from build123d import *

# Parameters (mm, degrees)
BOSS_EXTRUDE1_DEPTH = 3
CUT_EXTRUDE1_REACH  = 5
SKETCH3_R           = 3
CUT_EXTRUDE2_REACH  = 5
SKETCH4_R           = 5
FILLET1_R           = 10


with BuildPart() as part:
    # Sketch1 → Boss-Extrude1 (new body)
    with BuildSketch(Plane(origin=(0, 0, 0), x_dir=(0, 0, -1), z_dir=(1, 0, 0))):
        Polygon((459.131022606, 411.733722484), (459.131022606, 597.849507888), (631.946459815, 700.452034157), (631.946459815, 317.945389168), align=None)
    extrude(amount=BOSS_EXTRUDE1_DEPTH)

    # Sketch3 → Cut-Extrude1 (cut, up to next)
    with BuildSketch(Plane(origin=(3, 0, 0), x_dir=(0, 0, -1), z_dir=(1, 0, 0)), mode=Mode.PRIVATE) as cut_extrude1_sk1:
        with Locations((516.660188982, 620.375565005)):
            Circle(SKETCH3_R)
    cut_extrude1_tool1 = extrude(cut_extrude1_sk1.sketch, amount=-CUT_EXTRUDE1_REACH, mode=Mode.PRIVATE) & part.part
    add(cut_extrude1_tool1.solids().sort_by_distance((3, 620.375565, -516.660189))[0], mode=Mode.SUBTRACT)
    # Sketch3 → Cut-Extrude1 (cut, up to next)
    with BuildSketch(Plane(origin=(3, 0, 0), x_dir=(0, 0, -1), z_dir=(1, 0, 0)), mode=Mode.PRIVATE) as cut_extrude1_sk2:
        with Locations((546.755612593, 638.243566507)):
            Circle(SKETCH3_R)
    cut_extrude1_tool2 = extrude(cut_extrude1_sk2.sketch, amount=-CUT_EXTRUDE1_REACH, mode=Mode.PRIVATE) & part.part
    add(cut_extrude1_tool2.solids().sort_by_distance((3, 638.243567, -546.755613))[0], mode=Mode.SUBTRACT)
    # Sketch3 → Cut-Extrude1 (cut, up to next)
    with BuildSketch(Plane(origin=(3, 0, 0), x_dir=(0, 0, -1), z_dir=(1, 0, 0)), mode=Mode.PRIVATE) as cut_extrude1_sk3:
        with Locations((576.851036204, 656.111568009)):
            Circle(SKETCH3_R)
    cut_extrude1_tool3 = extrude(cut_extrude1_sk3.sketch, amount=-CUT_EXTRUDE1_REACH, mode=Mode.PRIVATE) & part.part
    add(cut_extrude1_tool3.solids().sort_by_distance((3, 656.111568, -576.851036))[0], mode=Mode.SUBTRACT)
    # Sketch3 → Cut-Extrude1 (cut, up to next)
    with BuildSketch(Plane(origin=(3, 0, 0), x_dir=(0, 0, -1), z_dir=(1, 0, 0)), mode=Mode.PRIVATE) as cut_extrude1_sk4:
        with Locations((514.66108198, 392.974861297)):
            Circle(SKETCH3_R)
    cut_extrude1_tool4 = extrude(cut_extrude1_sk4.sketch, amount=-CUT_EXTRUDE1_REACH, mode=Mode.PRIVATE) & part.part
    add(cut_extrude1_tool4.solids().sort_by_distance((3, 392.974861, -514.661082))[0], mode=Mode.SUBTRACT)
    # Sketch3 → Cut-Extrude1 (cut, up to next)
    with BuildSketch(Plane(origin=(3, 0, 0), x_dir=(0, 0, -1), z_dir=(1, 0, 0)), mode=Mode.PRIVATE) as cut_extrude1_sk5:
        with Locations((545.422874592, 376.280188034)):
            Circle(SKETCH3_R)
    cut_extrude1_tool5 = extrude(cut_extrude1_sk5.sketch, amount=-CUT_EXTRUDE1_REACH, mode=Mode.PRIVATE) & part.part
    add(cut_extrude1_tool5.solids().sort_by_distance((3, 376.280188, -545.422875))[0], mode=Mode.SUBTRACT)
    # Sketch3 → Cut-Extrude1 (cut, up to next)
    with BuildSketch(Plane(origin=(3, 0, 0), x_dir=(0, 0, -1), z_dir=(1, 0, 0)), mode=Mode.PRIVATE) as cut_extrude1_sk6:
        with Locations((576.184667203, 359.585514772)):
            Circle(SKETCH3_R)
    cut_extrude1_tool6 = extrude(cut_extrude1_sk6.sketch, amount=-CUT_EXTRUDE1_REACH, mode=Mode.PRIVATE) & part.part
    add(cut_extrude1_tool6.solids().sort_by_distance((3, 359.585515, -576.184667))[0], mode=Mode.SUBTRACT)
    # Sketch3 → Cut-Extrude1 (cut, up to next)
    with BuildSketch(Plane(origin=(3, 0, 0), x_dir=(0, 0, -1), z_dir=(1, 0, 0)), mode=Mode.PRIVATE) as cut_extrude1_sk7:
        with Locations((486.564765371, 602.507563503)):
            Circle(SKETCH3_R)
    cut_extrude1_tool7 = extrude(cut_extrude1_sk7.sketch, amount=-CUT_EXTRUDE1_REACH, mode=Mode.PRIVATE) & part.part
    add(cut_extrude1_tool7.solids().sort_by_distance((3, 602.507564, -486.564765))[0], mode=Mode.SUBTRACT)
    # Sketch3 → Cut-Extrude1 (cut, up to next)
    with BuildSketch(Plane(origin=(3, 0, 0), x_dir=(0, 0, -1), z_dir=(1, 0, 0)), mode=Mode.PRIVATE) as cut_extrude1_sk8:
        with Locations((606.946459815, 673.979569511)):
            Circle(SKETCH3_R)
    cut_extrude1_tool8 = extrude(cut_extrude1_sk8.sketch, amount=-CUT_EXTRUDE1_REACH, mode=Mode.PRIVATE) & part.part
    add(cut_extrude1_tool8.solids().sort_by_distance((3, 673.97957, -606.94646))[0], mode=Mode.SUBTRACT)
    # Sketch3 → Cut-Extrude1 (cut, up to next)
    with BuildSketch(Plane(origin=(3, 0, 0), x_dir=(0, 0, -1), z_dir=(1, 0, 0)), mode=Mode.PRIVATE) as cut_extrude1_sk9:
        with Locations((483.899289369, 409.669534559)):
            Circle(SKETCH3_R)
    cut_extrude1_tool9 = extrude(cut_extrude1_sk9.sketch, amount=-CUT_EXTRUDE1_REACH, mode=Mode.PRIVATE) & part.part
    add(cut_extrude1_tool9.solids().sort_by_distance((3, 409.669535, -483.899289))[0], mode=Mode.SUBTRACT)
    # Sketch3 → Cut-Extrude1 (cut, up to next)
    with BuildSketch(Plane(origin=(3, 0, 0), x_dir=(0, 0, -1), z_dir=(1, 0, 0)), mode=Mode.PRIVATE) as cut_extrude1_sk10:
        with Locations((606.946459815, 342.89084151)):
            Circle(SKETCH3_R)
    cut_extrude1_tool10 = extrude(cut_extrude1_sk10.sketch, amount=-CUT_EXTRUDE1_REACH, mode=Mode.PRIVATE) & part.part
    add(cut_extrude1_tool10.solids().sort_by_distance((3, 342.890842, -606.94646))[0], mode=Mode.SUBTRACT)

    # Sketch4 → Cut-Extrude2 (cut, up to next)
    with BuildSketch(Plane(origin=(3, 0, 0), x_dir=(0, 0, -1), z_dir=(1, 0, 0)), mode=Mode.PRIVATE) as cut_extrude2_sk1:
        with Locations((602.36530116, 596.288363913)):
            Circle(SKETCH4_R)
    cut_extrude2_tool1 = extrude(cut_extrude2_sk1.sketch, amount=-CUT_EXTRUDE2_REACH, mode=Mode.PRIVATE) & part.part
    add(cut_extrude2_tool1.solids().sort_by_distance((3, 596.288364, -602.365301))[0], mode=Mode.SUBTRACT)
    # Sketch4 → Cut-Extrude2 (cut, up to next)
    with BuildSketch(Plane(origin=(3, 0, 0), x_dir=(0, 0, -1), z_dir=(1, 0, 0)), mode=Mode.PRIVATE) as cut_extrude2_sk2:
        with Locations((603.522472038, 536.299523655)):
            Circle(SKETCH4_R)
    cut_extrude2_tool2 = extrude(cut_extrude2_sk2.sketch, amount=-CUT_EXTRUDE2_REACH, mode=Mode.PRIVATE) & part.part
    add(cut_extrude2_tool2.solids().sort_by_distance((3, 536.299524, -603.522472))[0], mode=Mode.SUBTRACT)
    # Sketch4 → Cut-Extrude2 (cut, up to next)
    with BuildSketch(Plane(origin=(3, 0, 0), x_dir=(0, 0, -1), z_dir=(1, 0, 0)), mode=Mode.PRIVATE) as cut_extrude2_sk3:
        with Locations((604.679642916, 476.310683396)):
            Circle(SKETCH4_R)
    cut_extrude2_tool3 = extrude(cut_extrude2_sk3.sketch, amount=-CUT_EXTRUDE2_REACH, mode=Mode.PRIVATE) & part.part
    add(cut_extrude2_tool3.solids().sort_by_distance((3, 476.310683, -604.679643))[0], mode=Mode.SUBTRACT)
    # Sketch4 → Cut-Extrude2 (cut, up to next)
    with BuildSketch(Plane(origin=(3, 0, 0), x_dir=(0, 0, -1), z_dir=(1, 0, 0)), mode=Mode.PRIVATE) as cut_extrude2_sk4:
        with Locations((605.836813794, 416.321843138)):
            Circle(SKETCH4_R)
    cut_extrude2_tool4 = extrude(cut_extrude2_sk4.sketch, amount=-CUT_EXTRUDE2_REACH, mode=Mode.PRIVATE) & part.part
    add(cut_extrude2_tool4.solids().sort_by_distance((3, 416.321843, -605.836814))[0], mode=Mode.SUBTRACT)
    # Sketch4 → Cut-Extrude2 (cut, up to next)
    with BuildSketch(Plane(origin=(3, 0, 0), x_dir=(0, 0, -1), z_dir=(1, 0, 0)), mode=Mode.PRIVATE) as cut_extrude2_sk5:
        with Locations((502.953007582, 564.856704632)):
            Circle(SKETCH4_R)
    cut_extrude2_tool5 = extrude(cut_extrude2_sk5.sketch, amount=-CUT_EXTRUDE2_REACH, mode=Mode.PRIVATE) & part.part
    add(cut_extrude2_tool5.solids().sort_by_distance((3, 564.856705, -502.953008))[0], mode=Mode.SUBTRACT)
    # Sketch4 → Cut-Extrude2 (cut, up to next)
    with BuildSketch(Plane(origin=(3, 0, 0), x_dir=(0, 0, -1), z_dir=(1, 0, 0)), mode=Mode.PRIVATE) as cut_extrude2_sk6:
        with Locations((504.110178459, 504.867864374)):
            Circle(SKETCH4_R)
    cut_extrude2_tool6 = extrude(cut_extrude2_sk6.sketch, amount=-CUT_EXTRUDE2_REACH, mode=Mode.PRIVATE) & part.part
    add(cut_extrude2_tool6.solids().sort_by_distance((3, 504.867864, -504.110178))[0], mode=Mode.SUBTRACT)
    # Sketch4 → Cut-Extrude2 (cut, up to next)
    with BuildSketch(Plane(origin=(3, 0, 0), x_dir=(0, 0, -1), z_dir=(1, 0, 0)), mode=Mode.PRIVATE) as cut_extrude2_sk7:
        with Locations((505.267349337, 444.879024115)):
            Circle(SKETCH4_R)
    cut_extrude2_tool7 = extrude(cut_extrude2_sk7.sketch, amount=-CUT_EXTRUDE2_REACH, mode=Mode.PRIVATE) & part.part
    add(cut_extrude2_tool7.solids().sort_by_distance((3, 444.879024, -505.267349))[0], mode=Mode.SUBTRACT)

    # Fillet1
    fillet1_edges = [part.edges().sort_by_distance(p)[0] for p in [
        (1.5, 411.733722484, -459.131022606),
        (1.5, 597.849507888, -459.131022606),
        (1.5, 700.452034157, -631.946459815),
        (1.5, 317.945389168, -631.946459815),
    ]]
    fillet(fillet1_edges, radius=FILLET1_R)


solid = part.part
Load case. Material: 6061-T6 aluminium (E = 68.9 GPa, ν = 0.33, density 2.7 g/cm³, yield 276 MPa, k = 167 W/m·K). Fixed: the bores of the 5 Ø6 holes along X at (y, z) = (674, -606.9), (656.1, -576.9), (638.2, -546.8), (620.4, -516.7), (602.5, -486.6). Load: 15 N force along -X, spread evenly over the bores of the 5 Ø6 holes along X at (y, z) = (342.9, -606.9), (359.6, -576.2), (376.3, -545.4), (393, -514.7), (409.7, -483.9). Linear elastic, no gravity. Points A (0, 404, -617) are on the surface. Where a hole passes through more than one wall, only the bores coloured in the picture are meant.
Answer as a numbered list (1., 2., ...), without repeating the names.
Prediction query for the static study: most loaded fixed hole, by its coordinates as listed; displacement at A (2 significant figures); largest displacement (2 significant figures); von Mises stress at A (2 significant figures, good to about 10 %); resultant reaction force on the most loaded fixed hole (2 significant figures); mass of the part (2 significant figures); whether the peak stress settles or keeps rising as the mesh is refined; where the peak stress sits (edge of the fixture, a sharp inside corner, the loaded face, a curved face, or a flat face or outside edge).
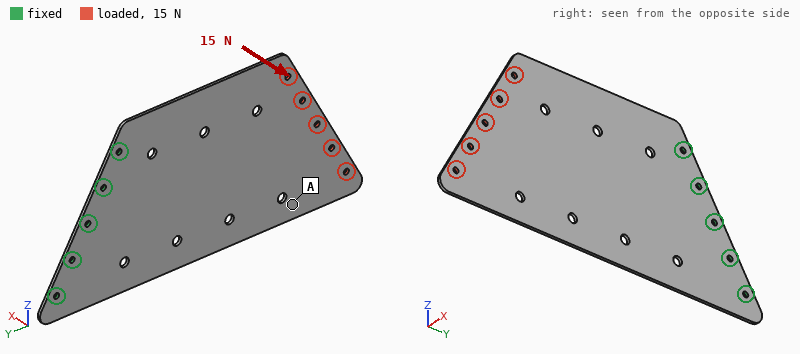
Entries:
1. (602.5, -486.6)
2. 2.4 mm
3. 3.8 mm
4. 2.4 MPa
5. 19 N
6. 390 g
7. keeps rising
8. edge of the fixture
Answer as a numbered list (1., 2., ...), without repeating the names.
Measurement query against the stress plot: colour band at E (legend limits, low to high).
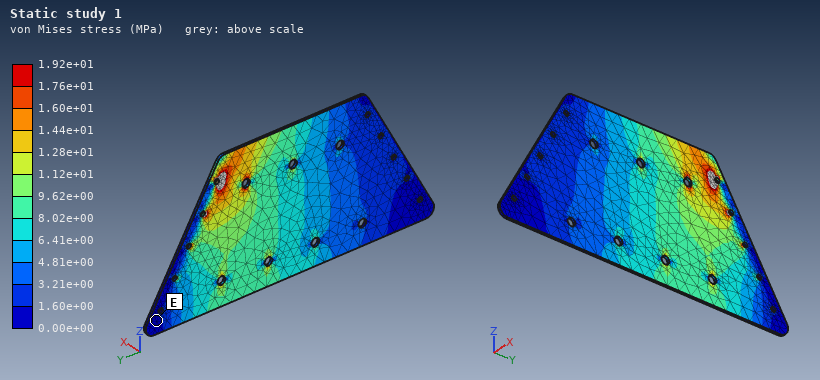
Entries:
1. 0.00e+00 to 1.60e+00 MPa
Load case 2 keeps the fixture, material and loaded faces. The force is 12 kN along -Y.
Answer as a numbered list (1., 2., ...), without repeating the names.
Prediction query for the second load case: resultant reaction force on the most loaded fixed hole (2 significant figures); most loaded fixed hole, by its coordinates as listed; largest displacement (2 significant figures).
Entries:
1. 3.0 kN
2. (602.5, -486.6)
3. 0.13 mm
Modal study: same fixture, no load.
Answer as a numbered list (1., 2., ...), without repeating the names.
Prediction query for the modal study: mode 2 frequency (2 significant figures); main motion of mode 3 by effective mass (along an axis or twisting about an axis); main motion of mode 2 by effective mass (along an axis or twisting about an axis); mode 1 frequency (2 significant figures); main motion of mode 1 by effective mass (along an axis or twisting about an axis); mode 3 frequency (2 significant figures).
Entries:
1. 130 Hz
2. along X
3. twisting about Y
4. 36 Hz
5. along X
6. 190 Hz
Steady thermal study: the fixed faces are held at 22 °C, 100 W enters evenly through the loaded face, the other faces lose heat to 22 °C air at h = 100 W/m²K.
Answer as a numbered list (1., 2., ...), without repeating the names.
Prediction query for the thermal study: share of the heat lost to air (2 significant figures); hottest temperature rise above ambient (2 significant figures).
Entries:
1. 99 %
2. 55 K
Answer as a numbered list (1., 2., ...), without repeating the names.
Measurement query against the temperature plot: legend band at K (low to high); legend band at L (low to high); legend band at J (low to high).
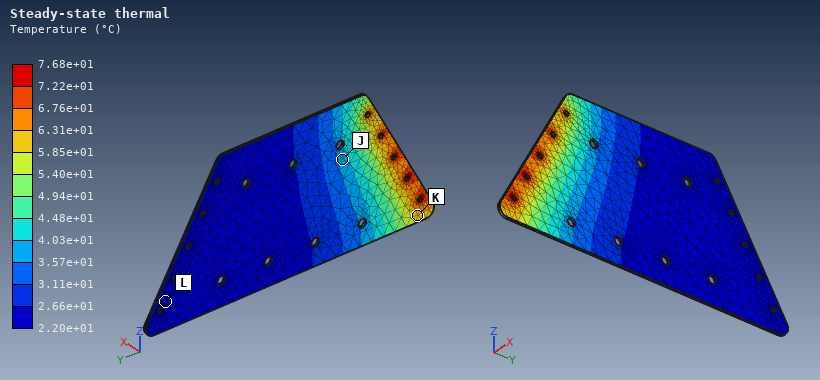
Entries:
1. 5.85e+01 to 6.31e+01 °C
2. 2.20e+01 to 2.66e+01 °C
3. 3.57e+01 to 4.03e+01 °C
